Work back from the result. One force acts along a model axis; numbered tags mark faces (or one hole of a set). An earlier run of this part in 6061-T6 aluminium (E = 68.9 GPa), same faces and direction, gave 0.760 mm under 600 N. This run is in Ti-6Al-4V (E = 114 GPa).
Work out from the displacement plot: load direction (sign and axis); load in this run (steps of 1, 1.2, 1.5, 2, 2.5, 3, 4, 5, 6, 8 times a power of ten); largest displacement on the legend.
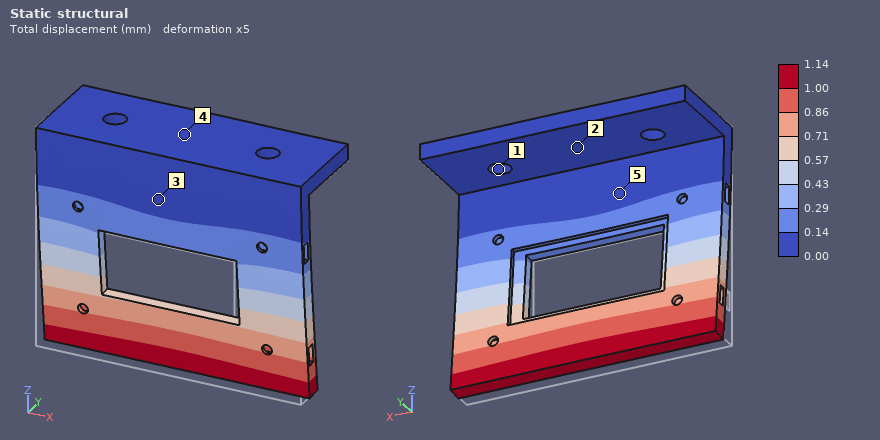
+Y
1.5 kN
1.14 mm
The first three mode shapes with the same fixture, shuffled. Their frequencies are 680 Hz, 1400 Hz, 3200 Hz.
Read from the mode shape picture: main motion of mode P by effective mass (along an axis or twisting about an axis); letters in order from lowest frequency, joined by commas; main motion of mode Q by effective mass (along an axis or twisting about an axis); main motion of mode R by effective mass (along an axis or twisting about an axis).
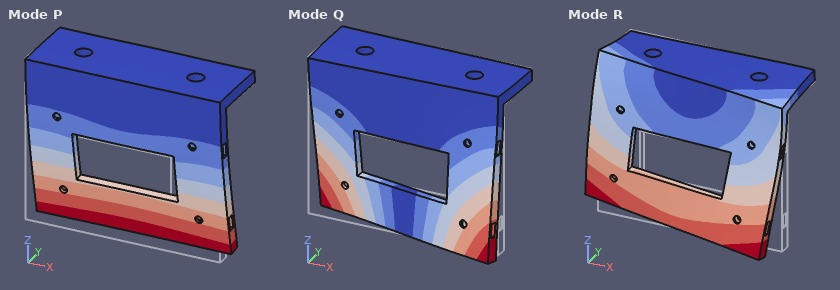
along Y
P, Q, R
twisting about Z
along X
